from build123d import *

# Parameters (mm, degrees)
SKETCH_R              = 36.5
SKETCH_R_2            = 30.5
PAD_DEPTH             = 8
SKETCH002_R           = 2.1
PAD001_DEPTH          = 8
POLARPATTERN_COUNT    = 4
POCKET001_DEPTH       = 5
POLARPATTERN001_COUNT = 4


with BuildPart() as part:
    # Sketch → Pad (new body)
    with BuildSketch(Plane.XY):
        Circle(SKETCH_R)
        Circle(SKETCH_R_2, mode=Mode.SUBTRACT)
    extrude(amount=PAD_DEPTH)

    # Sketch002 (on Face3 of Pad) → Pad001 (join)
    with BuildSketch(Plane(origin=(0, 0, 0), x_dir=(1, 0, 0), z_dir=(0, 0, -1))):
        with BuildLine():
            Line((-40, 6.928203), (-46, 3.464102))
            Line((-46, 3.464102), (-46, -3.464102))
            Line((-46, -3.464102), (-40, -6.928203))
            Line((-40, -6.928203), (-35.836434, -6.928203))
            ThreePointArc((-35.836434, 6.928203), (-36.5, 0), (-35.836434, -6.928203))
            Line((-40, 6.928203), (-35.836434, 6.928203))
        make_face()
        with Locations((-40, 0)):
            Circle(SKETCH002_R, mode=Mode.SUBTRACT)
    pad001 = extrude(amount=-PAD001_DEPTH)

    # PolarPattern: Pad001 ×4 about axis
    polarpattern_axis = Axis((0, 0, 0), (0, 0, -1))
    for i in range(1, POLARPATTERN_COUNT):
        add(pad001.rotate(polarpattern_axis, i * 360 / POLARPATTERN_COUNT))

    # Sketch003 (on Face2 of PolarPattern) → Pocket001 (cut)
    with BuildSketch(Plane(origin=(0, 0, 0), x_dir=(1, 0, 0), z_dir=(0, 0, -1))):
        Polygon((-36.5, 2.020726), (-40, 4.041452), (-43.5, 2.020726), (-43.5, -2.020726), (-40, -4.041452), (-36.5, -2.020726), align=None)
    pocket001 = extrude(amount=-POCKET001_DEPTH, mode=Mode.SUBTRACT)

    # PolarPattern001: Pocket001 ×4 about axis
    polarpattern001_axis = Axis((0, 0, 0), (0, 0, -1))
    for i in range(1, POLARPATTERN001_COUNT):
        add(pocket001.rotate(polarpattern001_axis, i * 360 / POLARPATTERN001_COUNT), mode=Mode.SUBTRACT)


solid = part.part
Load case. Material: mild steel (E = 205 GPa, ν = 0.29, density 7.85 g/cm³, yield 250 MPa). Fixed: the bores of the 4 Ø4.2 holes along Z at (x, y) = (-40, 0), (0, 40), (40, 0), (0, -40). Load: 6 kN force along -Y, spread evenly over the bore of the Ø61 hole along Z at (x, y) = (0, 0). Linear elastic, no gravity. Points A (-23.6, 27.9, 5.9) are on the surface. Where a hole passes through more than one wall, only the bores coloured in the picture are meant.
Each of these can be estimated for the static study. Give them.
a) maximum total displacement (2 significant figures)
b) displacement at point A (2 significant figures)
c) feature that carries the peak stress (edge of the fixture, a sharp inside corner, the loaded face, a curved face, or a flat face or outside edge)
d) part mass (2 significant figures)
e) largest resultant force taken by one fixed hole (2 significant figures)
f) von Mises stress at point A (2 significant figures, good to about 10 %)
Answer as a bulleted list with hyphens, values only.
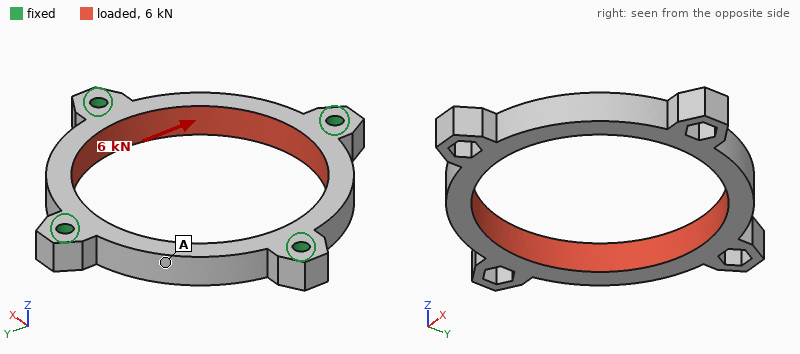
- 12 µm
- 9.3 µm
- edge of the fixture
- 100 g
- 2.1 kN
- 27 MPa
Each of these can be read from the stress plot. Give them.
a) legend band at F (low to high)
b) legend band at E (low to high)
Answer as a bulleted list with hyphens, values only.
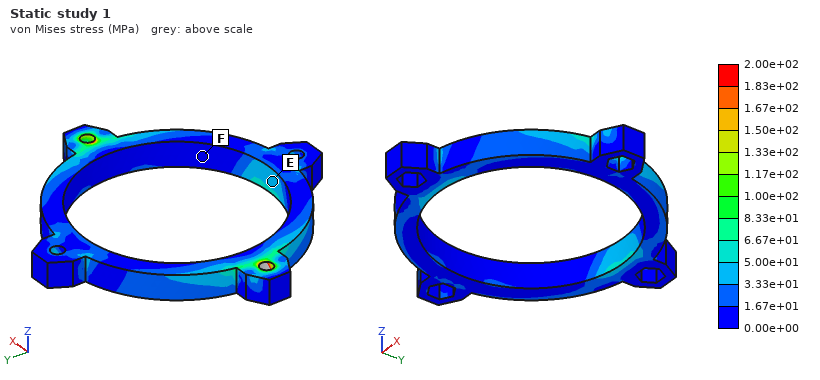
- 0.00e+00 to 1.67e+01 MPa
- 3.33e+01 to 5.00e+01 MPa
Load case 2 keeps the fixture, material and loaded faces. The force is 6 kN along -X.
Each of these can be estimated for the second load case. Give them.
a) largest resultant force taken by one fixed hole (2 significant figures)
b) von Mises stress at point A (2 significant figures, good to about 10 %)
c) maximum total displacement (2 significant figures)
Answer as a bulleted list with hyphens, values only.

- 2.1 kN
- 32 MPa
- 12 µm
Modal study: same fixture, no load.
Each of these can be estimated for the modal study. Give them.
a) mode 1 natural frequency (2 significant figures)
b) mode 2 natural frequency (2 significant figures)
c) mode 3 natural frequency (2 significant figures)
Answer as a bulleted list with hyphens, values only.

- 7600 Hz
- 9200 Hz
- 9200 Hz
